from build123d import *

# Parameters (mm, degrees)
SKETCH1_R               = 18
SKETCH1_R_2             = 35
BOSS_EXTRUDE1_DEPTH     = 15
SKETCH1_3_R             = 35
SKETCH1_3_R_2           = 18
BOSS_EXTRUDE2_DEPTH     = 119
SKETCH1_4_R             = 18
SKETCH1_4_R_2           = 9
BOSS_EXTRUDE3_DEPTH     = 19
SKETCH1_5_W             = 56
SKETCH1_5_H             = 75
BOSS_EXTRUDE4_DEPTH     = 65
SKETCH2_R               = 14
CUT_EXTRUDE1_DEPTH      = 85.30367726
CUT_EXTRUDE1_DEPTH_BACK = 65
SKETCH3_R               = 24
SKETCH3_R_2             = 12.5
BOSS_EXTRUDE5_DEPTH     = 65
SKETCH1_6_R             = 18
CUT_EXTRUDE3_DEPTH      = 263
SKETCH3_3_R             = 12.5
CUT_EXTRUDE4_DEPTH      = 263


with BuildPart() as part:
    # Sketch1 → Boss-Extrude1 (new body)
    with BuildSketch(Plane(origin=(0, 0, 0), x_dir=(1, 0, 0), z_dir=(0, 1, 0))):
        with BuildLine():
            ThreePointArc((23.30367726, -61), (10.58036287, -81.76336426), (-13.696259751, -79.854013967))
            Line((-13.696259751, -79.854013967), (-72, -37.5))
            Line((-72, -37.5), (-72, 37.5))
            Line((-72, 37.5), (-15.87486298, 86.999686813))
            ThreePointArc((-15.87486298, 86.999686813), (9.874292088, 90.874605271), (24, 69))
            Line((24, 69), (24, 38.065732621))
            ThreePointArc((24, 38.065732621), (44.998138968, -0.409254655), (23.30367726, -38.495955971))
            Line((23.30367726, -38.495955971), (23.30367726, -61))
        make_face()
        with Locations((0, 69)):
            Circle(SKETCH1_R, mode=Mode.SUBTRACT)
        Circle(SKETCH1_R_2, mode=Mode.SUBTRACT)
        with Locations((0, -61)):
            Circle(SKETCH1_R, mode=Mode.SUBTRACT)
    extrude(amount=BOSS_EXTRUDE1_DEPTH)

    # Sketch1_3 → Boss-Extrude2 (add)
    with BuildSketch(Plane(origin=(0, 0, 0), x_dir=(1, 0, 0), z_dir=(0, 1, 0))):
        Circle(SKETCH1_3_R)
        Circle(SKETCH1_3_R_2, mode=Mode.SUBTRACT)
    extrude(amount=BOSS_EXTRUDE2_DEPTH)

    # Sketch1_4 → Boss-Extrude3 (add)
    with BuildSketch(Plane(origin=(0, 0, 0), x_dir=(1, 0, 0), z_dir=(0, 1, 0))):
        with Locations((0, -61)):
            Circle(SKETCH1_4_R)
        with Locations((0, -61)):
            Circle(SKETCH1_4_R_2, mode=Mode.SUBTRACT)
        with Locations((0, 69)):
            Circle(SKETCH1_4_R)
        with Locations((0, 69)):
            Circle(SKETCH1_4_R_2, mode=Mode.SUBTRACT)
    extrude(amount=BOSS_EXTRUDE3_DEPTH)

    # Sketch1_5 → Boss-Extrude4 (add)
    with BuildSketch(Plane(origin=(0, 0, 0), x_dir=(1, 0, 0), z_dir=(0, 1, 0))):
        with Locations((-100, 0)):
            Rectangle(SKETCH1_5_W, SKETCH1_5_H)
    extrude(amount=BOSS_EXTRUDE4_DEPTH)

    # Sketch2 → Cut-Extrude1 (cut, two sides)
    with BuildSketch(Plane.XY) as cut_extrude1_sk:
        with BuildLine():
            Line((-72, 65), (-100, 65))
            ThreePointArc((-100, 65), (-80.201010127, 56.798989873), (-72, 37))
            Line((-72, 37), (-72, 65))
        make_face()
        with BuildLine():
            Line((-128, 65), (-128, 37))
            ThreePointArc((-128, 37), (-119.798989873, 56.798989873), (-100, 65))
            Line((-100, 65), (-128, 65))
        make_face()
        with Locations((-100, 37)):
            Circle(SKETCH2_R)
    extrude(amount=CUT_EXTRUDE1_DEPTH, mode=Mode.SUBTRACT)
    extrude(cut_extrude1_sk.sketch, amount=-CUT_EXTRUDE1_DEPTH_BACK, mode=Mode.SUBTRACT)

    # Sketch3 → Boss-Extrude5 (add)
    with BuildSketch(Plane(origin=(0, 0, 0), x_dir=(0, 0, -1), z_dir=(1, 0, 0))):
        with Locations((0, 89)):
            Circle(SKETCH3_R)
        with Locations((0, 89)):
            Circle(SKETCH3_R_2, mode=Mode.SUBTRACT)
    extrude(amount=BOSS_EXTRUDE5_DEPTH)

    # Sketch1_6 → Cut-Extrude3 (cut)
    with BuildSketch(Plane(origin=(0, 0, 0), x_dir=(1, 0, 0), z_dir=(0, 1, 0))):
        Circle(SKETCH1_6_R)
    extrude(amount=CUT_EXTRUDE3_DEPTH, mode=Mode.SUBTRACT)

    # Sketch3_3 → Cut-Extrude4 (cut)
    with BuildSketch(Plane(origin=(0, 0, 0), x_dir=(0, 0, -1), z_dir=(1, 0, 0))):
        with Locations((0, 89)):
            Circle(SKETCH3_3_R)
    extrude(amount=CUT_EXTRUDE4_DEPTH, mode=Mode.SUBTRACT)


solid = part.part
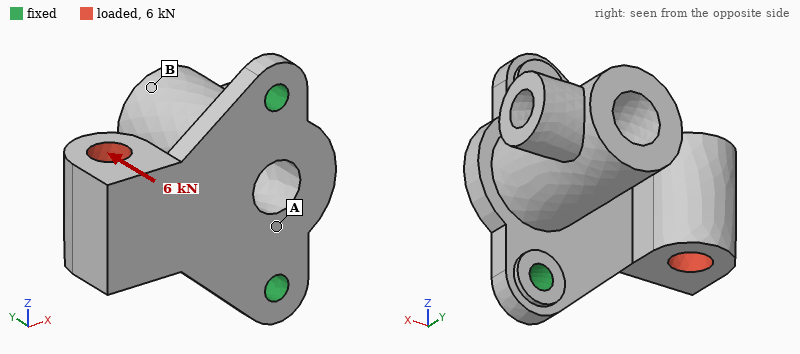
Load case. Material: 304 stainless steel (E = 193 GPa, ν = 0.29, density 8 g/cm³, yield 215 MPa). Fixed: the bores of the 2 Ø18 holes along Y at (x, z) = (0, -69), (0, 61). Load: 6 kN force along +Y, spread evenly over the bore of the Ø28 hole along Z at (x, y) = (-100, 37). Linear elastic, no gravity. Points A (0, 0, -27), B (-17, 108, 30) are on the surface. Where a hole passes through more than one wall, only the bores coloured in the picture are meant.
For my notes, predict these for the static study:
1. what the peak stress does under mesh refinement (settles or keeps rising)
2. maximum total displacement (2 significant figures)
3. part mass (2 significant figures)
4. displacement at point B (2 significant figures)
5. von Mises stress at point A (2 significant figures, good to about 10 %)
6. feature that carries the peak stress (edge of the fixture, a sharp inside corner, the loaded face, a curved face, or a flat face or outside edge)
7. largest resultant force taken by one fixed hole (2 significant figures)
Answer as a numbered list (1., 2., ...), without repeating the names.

1. keeps rising
2. 0.41 mm
3. 5.9 kg
4. 0.12 mm
5. 30 MPa
6. edge of the fixture
7. 3.3 kN
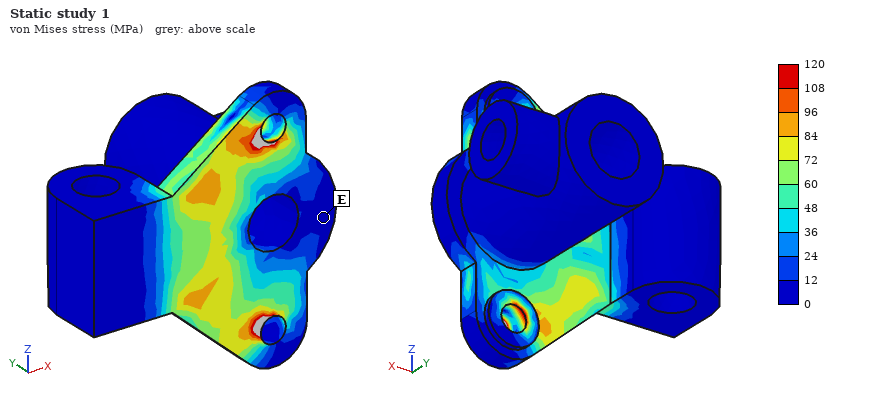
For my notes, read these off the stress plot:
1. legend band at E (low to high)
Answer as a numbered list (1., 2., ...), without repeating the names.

1. 0 to 12 MPa
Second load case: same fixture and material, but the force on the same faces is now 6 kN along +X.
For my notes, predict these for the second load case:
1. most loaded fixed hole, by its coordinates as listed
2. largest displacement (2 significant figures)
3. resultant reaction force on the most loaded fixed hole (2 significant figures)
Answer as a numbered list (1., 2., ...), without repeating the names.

1. (0, 61)
2. 0.20 mm
3. 3.4 kN
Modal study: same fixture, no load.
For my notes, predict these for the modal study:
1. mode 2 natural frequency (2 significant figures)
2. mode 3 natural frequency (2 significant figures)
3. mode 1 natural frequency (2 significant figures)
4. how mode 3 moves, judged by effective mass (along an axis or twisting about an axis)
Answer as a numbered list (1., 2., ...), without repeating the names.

1. 1000 Hz
2. 1600 Hz
3. 480 Hz
4. along Z
